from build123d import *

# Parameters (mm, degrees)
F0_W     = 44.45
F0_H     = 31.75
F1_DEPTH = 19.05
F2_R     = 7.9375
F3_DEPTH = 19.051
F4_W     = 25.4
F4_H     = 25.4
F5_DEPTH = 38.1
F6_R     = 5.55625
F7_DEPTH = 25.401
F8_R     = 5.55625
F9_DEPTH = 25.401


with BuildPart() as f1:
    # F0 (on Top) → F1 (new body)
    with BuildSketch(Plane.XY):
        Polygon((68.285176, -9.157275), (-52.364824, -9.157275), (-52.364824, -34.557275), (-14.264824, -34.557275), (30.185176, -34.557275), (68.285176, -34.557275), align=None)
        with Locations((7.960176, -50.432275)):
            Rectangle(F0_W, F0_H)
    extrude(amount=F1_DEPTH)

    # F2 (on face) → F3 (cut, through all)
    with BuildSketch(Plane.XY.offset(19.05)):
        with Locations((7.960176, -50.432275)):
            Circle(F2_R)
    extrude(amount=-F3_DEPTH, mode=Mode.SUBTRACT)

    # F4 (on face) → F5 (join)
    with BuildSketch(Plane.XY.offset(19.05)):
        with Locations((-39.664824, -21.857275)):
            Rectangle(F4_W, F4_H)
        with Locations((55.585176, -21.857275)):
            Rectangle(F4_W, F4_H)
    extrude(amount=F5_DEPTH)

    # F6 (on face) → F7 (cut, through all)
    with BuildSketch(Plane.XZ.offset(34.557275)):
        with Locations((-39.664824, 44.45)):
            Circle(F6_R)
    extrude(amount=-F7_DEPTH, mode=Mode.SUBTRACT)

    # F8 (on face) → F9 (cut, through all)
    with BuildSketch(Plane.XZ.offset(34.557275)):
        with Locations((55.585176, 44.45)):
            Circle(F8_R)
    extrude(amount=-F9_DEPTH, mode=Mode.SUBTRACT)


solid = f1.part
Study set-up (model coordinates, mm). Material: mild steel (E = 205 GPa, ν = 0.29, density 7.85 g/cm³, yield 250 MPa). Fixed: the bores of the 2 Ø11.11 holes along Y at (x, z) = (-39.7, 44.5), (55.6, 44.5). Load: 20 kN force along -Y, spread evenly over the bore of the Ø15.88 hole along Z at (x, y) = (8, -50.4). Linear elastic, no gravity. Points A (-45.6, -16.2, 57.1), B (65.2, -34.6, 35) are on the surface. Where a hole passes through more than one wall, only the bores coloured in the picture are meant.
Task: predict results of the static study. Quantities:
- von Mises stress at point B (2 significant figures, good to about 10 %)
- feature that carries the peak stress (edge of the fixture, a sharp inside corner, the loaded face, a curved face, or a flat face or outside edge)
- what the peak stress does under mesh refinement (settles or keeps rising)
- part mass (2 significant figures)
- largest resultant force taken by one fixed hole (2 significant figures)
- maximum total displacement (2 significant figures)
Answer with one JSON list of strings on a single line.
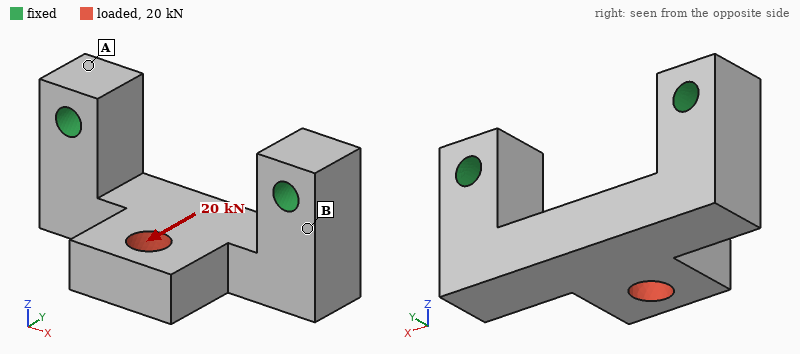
["71 MPa", "edge of the fixture", "keeps rising", "990 g", "10 kN", "70 µm"]
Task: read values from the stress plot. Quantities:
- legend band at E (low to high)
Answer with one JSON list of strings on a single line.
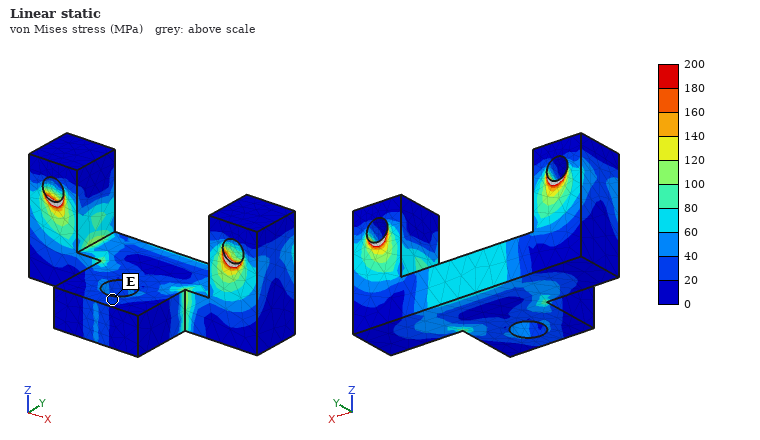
["20 to 40 MPa"]
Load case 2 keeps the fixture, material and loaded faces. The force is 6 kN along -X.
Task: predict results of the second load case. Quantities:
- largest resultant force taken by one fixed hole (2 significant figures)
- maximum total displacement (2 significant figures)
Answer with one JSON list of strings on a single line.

["3.6 kN", "20 µm"]
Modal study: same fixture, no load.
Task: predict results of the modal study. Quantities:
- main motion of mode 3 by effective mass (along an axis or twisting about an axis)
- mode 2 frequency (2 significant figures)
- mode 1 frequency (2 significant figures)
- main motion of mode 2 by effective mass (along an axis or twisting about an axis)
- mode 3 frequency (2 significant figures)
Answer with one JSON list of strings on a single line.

["along X", "5300 Hz", "3600 Hz", "along Y", "5600 Hz"]
